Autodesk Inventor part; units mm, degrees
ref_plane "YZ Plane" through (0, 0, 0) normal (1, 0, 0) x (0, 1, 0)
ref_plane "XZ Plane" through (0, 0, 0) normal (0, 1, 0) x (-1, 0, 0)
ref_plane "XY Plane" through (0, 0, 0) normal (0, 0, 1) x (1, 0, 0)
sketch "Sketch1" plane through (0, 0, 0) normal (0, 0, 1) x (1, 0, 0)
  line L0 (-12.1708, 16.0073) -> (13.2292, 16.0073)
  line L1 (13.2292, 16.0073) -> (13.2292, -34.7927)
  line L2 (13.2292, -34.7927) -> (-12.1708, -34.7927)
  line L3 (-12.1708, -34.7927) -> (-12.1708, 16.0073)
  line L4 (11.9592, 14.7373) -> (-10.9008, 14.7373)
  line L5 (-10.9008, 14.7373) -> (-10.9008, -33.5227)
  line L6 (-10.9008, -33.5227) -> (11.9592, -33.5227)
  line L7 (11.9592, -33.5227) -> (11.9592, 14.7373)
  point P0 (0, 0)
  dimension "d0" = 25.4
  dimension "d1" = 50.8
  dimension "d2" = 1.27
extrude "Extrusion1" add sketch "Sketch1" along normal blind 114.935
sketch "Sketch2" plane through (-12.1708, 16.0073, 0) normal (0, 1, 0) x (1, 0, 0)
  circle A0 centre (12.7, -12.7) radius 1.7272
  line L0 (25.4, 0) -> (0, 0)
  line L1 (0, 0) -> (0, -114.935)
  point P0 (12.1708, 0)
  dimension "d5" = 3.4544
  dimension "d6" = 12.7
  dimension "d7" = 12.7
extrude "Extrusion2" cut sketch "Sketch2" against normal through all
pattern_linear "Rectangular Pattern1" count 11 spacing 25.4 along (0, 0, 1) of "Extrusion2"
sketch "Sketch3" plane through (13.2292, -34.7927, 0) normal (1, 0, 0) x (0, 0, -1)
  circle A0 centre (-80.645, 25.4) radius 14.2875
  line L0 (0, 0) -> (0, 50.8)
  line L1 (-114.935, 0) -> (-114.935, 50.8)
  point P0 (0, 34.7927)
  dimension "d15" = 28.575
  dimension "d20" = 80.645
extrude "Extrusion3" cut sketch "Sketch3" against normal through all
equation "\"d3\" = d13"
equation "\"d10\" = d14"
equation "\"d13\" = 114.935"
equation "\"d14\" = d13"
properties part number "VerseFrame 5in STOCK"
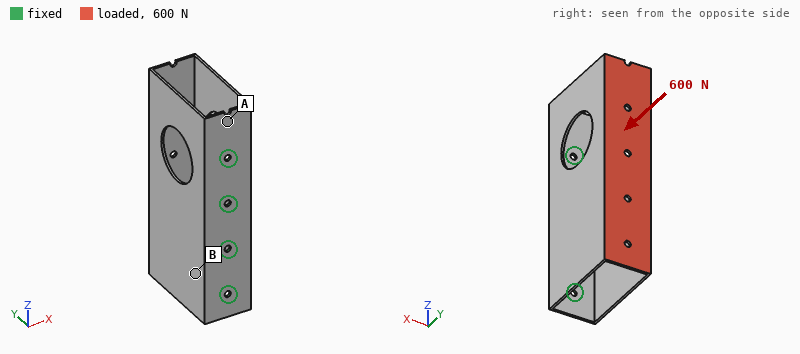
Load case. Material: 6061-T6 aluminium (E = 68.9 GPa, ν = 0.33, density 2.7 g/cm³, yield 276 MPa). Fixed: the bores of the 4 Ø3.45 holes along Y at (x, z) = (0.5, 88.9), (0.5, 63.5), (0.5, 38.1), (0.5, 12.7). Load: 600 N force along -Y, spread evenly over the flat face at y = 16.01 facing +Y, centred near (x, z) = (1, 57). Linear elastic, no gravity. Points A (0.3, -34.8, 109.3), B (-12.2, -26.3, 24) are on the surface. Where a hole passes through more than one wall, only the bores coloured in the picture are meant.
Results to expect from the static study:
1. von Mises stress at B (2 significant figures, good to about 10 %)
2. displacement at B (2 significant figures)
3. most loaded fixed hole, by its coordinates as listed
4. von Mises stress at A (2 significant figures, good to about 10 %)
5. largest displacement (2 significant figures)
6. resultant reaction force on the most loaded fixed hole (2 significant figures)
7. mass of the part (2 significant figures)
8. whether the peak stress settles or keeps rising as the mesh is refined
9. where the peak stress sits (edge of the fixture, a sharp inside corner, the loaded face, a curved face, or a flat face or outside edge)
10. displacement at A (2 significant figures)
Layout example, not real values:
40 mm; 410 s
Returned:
14 MPa; 0.096 mm; (0.5, 88.9); 36 MPa; 0.20 mm; 200 N; 53 g; keeps rising; edge of the fixture; 0.081 mm
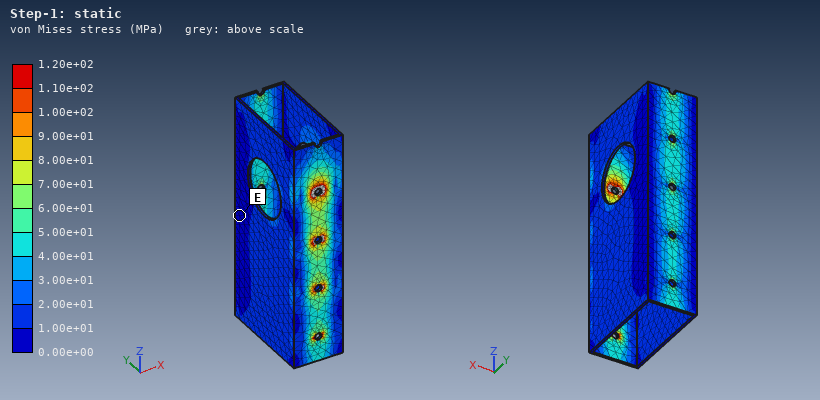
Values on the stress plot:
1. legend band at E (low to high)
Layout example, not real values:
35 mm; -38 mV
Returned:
0.00e+00 to 1.00e+01 MPa
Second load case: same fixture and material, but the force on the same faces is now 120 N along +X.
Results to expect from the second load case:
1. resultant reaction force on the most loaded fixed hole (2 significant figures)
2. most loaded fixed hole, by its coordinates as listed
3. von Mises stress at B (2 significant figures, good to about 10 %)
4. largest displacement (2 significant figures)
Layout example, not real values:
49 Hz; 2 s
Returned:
49 N; (0.5, 88.9); 30 MPa; 1.5 mm
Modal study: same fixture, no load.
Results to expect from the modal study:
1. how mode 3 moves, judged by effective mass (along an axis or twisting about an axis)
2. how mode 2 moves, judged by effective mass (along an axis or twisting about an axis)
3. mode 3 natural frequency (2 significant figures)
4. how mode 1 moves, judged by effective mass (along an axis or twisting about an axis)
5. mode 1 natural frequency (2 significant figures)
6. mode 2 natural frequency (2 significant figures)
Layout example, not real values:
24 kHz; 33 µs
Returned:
along Z; twisting about Y; 1200 Hz; along X; 310 Hz; 990 Hz
